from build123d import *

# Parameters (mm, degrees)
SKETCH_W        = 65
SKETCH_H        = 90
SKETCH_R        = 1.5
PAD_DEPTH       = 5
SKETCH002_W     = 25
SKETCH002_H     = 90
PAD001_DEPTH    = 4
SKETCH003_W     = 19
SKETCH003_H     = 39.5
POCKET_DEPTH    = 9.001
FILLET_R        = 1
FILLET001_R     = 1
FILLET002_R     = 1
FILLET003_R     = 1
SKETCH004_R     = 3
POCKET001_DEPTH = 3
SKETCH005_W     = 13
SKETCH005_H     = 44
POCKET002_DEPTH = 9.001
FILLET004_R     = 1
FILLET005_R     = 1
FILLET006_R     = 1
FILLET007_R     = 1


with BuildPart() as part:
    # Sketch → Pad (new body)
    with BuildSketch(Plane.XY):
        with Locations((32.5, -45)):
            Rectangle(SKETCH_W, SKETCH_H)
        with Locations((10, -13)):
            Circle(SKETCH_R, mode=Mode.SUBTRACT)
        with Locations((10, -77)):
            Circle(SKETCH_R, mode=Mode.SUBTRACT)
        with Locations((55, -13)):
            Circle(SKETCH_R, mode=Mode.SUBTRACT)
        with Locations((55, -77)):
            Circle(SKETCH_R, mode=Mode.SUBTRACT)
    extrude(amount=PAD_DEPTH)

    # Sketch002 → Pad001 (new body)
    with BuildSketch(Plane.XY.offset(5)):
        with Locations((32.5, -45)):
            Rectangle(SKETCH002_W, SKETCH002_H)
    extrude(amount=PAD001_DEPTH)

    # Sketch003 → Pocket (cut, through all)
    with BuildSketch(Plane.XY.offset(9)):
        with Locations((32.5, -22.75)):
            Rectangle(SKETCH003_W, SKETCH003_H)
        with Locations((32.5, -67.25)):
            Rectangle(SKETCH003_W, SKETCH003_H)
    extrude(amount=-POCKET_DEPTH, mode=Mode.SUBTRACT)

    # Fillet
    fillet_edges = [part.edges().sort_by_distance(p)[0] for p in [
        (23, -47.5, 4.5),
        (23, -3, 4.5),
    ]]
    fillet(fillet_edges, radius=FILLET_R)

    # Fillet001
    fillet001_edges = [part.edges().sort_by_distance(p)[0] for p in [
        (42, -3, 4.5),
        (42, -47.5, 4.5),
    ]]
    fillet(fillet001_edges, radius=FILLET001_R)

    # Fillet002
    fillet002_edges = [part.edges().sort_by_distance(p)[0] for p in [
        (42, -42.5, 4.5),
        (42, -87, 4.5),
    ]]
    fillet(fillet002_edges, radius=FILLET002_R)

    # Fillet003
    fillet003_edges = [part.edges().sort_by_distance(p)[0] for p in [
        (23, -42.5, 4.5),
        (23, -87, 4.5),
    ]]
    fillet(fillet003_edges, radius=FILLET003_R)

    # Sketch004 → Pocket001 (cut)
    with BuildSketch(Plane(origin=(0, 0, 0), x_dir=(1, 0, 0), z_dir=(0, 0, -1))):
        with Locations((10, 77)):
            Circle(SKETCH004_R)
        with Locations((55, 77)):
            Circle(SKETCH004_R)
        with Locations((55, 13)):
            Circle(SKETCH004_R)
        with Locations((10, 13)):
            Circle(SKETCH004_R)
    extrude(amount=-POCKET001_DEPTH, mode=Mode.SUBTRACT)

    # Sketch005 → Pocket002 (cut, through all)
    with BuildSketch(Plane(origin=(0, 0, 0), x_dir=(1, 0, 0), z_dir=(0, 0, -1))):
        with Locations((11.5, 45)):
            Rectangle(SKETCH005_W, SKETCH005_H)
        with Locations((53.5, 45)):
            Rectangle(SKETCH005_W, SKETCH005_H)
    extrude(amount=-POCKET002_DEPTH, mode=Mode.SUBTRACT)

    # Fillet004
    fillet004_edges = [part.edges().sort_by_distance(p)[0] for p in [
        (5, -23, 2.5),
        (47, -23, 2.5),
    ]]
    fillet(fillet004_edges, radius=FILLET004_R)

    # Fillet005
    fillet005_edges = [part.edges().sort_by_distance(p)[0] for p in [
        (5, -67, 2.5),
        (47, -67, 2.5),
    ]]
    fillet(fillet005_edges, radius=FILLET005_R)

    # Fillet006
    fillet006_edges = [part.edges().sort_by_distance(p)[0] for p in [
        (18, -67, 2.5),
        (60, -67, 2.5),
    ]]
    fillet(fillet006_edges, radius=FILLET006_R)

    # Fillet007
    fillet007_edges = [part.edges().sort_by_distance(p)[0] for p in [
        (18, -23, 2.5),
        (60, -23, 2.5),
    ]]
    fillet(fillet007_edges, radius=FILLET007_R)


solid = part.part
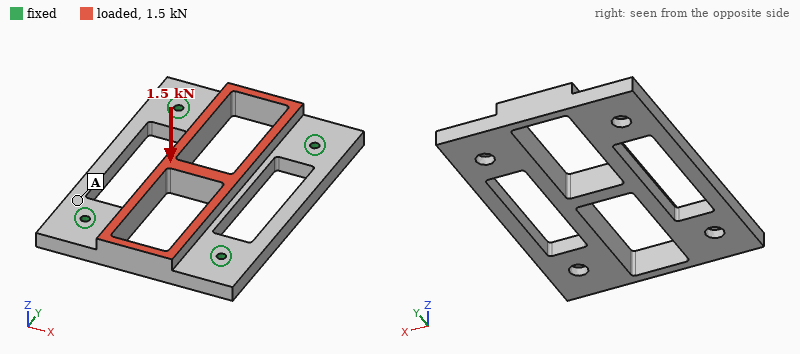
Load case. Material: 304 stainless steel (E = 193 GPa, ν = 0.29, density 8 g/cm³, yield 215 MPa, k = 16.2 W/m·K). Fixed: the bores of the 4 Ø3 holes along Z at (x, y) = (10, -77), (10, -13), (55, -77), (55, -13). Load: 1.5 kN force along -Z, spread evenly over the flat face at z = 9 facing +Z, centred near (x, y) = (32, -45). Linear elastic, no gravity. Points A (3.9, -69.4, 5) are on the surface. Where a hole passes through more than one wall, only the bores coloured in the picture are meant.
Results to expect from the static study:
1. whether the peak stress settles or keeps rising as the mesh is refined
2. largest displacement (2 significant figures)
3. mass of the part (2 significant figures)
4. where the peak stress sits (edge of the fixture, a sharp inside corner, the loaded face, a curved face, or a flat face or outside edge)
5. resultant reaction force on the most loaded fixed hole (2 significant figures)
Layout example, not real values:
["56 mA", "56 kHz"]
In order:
["keeps rising", "31 µm", "150 g", "edge of the fixture", "380 N"]
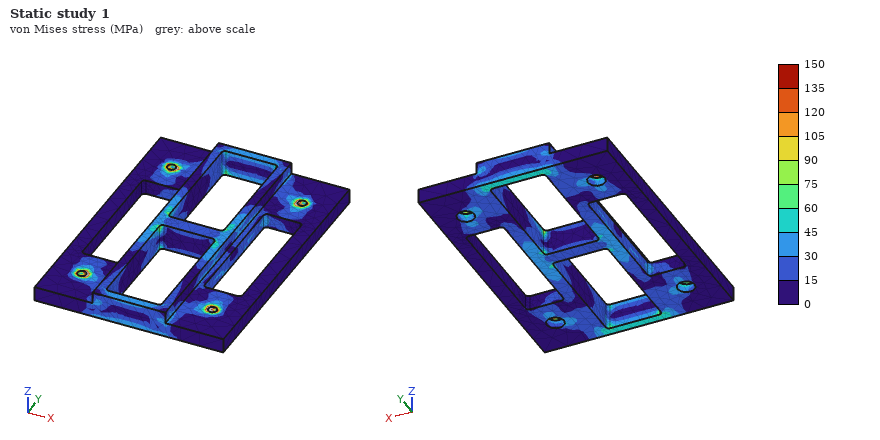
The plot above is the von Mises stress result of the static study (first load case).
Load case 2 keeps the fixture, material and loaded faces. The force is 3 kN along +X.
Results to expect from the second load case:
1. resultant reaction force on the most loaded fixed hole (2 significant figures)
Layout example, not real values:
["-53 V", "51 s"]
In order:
["790 N"]
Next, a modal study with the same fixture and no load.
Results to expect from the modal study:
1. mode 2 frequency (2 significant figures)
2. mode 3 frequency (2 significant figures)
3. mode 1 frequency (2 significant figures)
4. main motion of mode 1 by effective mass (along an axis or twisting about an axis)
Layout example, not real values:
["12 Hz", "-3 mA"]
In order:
["5200 Hz", "5500 Hz", "4300 Hz", "along Z"]
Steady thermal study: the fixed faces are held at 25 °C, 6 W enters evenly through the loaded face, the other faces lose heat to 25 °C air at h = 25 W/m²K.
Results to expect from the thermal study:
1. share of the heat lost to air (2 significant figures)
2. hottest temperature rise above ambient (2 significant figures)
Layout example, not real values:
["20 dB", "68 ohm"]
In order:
["43 %", "26 K"]
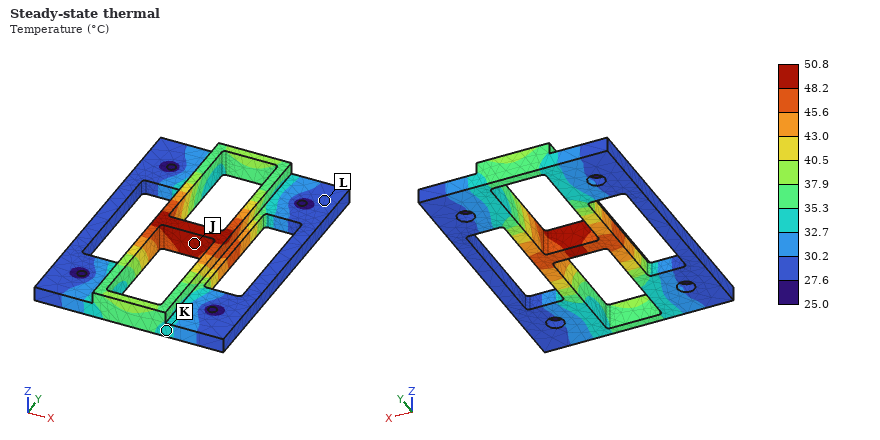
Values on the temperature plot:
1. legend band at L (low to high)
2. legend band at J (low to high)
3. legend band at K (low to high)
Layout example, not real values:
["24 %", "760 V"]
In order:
["27.6 to 30.2 °C", "48.2 to 50.8 °C", "32.7 to 35.3 °C"]
